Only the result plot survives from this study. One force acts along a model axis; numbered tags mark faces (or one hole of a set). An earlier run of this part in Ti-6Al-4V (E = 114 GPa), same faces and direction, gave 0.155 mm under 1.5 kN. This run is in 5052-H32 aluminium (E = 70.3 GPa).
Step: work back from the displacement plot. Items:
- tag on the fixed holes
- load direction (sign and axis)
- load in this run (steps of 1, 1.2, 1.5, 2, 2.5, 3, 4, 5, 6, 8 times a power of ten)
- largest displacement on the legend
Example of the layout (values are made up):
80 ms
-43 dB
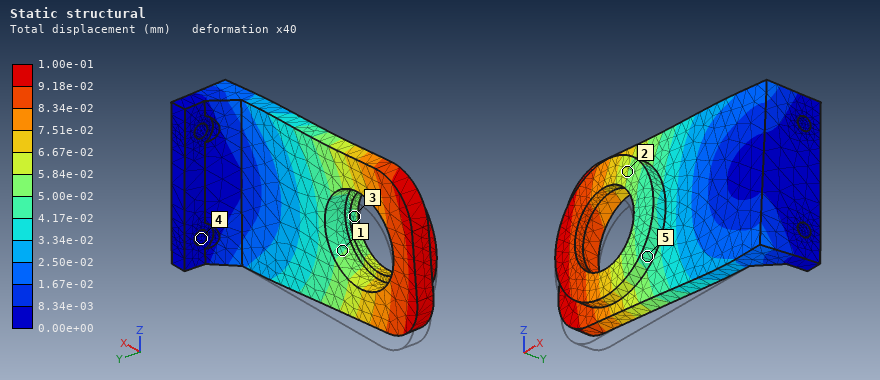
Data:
4
+Z
600 N
1.00e-01 mm
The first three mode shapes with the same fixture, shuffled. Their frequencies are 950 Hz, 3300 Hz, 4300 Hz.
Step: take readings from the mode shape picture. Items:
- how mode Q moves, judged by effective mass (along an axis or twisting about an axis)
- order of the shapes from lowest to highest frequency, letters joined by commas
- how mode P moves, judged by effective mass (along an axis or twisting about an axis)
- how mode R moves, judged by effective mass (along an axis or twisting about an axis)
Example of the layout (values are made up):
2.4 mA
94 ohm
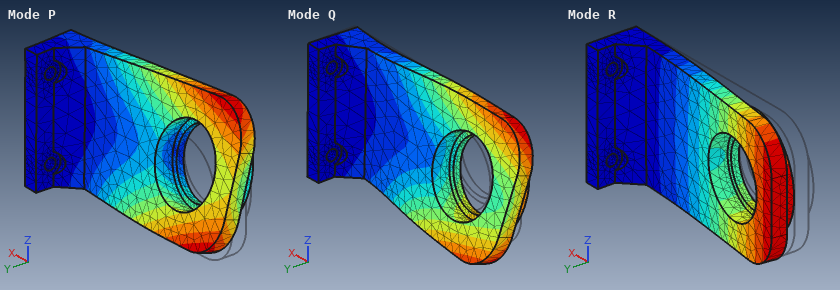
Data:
along Z
R, P, Q
along Z
along Y
